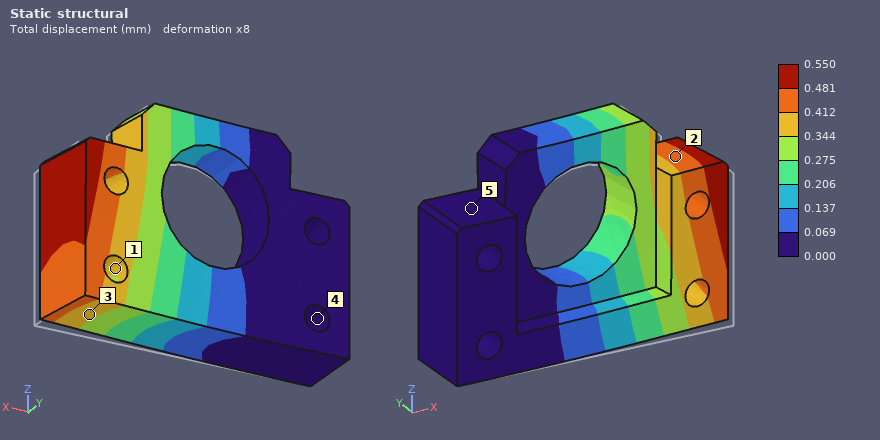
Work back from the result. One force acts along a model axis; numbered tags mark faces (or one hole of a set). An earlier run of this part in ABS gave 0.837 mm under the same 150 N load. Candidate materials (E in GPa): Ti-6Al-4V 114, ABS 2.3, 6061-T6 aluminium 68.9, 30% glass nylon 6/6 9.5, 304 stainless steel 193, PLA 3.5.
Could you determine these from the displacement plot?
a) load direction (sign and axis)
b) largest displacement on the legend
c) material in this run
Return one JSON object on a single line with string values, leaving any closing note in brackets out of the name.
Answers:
{"load direction": "+Y", "largest displacement on the legend": "0.550 mm", "material in this run": "PLA"}
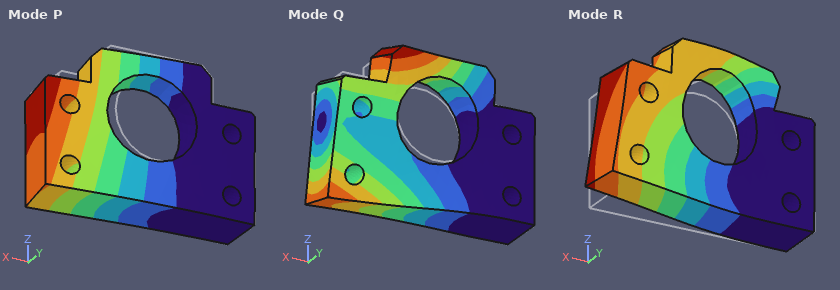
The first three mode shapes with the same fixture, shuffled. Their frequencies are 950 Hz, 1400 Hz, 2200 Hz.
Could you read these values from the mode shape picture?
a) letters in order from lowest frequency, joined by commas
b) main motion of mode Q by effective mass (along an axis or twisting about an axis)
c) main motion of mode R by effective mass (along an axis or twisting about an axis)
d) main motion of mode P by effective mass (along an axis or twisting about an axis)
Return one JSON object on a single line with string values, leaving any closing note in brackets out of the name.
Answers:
{"letters in order from lowest frequency, joined by commas": "P, R, Q", "main motion of mode Q by effective mass": "twisting about X", "main motion of mode R by effective mass": "along Z", "main motion of mode P by effective mass": "along Y"}
